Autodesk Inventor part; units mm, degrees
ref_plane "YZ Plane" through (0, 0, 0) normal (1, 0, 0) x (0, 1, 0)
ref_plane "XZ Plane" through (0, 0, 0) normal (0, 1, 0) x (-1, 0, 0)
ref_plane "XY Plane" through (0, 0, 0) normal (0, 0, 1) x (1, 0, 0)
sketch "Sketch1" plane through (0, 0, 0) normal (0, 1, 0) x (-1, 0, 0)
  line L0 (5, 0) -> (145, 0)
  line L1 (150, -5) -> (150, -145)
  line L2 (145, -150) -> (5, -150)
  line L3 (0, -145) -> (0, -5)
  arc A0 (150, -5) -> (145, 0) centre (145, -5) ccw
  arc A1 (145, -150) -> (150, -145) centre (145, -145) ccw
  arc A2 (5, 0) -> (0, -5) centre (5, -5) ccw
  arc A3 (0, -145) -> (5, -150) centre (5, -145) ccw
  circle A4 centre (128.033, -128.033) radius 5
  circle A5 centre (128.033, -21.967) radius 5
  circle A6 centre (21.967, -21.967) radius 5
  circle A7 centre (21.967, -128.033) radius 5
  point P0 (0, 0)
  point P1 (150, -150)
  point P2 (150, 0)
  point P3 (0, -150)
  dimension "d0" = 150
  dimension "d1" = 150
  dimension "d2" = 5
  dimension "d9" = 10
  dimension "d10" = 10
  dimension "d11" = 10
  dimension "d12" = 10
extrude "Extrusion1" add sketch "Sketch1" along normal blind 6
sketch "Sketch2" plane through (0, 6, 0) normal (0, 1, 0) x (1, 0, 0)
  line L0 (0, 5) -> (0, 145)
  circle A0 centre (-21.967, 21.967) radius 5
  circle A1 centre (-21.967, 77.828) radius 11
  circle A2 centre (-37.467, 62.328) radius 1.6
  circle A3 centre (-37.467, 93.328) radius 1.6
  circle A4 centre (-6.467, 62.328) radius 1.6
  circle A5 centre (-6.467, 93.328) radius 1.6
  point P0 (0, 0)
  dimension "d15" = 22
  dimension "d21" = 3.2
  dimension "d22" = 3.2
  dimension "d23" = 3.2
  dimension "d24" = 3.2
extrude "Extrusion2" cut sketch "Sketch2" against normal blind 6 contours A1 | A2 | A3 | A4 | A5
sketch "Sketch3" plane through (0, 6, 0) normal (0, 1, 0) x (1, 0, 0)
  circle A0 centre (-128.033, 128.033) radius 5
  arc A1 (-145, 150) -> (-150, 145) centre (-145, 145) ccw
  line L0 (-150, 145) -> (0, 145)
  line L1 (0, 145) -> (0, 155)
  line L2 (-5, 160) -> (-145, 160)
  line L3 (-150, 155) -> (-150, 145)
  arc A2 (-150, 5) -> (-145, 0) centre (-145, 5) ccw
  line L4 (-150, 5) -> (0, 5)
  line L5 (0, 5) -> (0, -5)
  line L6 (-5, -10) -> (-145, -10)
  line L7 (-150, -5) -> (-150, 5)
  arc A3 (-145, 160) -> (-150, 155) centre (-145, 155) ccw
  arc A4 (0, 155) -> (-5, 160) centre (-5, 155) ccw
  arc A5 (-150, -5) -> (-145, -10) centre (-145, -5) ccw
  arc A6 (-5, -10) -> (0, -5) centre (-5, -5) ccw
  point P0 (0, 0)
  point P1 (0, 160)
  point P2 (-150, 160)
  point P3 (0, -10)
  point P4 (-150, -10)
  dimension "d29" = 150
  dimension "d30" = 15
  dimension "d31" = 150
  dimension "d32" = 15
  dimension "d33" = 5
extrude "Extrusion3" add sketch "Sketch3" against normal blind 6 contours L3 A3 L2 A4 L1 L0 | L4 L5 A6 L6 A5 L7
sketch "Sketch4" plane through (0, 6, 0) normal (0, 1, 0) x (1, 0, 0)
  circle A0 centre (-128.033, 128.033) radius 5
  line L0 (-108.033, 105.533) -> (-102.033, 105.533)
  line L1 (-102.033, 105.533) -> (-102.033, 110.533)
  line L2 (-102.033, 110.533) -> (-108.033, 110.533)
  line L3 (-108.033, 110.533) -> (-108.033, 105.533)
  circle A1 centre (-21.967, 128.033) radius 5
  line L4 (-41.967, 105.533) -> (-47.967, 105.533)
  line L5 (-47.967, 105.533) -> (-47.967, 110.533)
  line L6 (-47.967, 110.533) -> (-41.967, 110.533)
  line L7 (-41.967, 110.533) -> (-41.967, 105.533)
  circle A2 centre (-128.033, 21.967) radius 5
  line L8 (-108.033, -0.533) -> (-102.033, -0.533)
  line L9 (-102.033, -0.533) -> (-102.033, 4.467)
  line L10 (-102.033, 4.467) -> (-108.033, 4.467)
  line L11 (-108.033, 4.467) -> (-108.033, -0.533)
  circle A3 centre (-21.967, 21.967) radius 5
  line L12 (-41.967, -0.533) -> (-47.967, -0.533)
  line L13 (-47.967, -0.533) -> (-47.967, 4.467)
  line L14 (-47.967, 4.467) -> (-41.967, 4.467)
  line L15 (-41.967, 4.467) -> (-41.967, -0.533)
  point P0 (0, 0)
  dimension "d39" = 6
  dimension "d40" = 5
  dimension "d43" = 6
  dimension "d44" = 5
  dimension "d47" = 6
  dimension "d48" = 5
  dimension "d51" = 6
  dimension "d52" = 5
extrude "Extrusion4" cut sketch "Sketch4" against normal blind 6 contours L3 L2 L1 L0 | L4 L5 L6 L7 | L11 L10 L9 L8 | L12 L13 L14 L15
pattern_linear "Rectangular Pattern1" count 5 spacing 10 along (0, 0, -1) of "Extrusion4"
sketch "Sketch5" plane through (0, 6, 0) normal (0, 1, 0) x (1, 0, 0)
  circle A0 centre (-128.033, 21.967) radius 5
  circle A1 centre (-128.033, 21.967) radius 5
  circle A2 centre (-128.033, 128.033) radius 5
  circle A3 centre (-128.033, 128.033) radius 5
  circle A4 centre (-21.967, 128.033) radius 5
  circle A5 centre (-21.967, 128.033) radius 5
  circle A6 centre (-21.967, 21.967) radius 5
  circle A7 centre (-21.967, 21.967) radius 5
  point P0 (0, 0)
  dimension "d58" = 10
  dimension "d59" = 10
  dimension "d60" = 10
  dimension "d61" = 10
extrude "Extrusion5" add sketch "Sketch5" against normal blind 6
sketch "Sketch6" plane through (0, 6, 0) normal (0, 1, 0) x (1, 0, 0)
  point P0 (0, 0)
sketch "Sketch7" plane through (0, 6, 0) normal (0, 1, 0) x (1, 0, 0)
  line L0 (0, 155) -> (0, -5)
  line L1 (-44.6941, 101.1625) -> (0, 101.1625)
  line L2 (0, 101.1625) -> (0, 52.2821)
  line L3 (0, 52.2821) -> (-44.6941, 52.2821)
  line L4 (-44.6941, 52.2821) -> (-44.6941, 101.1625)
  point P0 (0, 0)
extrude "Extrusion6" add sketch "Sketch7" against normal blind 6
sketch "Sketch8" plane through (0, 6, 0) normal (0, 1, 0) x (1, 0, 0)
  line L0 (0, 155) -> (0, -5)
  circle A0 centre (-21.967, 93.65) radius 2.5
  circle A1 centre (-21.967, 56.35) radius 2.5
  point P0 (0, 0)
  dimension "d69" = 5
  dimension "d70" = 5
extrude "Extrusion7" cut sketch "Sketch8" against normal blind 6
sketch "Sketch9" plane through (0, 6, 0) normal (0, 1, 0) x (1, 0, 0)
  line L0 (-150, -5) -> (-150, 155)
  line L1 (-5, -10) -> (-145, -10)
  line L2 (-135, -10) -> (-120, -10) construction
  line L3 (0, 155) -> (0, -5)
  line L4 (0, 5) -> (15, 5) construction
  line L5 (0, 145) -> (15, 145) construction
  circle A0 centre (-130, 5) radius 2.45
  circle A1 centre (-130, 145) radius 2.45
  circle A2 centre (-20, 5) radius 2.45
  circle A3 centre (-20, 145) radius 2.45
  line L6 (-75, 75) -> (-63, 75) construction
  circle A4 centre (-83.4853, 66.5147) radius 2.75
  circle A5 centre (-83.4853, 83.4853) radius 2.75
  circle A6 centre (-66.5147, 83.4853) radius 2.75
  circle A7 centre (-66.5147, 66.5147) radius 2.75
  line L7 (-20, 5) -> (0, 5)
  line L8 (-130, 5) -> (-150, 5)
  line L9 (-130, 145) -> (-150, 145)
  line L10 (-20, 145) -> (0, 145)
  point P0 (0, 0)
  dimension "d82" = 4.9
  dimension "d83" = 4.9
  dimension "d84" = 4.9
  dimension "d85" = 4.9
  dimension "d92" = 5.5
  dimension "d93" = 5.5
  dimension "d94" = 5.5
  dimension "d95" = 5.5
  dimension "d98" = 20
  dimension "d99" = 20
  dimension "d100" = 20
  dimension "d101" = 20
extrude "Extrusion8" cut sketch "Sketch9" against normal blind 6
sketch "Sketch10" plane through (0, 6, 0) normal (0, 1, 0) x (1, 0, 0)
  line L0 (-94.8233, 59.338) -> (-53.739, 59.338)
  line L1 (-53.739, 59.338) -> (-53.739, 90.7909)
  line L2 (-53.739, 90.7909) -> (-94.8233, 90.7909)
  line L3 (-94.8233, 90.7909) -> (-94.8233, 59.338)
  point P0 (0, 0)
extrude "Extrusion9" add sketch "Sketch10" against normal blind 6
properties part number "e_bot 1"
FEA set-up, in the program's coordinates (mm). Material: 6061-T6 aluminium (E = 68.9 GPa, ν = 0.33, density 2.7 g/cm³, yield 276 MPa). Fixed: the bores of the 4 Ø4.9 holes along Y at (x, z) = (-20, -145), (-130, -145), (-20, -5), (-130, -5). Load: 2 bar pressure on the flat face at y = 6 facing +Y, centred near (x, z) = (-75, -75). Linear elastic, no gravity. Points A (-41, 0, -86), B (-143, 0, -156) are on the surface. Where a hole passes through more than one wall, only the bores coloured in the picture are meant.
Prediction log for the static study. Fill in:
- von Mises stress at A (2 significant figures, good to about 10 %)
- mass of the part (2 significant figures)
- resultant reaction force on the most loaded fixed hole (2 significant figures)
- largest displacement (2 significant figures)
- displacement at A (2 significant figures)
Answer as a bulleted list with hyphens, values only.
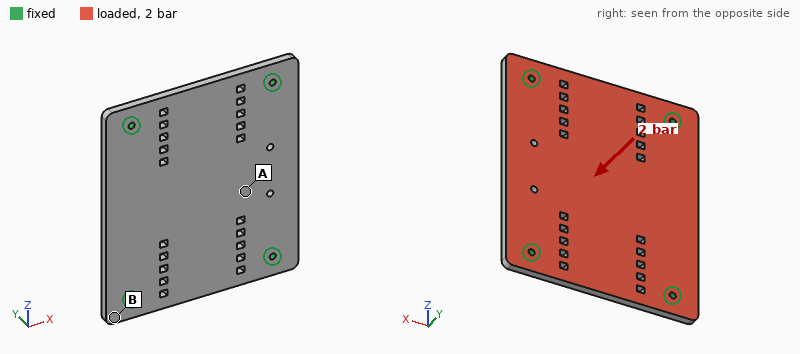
- 29 MPa
- 400 g
- 1.2 kN
- 0.31 mm
- 0.27 mm
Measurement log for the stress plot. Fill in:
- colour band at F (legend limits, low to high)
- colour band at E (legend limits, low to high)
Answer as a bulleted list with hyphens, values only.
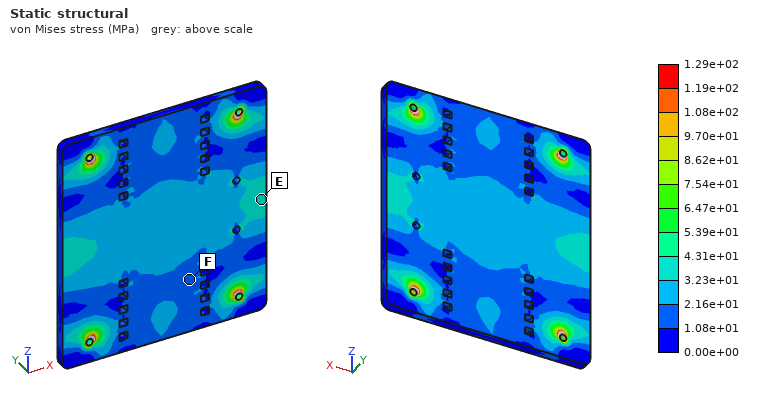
- 1.08e+01 to 2.16e+01 MPa
- 3.23e+01 to 4.31e+01 MPa
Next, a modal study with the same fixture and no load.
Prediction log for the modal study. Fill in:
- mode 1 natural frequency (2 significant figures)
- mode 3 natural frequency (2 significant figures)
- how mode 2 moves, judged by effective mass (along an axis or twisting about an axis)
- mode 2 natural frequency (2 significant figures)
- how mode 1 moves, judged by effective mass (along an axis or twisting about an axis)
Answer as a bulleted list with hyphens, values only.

- 1200 Hz
- 2200 Hz
- twisting about Z
- 1700 Hz
- along Y
